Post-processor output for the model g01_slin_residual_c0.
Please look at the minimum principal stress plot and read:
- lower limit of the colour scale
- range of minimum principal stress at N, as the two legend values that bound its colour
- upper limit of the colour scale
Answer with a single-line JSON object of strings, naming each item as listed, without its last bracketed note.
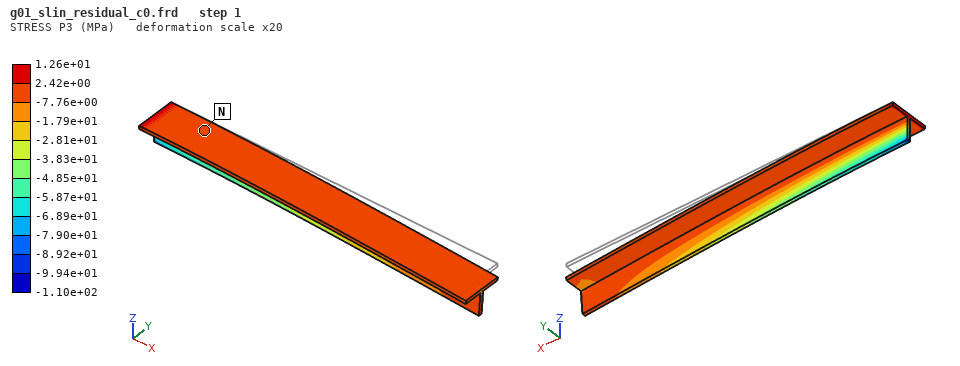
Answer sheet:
{"lower limit of the colour scale": "-1.10e+02 MPa", "range of minimum principal stress at N, as the two legend values that bound its colour": "-7.76e+00 to 2.42e+00 MPa", "upper limit of the colour scale": "1.26e+01 MPa"}
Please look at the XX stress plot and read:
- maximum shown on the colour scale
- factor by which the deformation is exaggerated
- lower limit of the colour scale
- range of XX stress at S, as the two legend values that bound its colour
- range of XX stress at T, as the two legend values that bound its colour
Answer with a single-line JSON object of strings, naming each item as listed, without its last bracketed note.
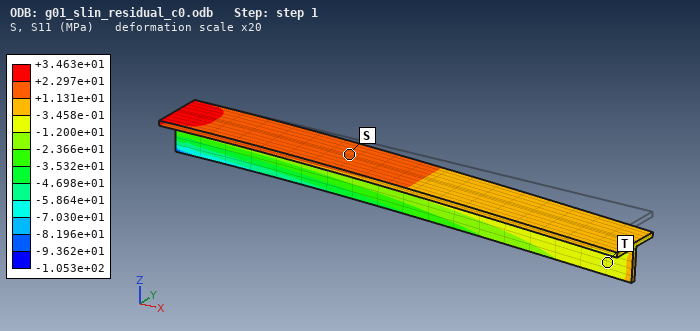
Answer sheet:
{"maximum shown on the colour scale": "+3.463e+01 MPa", "factor by which the deformation is exaggerated": "20", "lower limit of the colour scale": "-1.053e+02 MPa", "range of XX stress at S, as the two legend values that bound its colour": "+1.131e+01 to +2.297e+01 MPa", "range of XX stress at T, as the two legend values that bound its colour": "-1.200e+01 to -3.458e-01 MPa"}
